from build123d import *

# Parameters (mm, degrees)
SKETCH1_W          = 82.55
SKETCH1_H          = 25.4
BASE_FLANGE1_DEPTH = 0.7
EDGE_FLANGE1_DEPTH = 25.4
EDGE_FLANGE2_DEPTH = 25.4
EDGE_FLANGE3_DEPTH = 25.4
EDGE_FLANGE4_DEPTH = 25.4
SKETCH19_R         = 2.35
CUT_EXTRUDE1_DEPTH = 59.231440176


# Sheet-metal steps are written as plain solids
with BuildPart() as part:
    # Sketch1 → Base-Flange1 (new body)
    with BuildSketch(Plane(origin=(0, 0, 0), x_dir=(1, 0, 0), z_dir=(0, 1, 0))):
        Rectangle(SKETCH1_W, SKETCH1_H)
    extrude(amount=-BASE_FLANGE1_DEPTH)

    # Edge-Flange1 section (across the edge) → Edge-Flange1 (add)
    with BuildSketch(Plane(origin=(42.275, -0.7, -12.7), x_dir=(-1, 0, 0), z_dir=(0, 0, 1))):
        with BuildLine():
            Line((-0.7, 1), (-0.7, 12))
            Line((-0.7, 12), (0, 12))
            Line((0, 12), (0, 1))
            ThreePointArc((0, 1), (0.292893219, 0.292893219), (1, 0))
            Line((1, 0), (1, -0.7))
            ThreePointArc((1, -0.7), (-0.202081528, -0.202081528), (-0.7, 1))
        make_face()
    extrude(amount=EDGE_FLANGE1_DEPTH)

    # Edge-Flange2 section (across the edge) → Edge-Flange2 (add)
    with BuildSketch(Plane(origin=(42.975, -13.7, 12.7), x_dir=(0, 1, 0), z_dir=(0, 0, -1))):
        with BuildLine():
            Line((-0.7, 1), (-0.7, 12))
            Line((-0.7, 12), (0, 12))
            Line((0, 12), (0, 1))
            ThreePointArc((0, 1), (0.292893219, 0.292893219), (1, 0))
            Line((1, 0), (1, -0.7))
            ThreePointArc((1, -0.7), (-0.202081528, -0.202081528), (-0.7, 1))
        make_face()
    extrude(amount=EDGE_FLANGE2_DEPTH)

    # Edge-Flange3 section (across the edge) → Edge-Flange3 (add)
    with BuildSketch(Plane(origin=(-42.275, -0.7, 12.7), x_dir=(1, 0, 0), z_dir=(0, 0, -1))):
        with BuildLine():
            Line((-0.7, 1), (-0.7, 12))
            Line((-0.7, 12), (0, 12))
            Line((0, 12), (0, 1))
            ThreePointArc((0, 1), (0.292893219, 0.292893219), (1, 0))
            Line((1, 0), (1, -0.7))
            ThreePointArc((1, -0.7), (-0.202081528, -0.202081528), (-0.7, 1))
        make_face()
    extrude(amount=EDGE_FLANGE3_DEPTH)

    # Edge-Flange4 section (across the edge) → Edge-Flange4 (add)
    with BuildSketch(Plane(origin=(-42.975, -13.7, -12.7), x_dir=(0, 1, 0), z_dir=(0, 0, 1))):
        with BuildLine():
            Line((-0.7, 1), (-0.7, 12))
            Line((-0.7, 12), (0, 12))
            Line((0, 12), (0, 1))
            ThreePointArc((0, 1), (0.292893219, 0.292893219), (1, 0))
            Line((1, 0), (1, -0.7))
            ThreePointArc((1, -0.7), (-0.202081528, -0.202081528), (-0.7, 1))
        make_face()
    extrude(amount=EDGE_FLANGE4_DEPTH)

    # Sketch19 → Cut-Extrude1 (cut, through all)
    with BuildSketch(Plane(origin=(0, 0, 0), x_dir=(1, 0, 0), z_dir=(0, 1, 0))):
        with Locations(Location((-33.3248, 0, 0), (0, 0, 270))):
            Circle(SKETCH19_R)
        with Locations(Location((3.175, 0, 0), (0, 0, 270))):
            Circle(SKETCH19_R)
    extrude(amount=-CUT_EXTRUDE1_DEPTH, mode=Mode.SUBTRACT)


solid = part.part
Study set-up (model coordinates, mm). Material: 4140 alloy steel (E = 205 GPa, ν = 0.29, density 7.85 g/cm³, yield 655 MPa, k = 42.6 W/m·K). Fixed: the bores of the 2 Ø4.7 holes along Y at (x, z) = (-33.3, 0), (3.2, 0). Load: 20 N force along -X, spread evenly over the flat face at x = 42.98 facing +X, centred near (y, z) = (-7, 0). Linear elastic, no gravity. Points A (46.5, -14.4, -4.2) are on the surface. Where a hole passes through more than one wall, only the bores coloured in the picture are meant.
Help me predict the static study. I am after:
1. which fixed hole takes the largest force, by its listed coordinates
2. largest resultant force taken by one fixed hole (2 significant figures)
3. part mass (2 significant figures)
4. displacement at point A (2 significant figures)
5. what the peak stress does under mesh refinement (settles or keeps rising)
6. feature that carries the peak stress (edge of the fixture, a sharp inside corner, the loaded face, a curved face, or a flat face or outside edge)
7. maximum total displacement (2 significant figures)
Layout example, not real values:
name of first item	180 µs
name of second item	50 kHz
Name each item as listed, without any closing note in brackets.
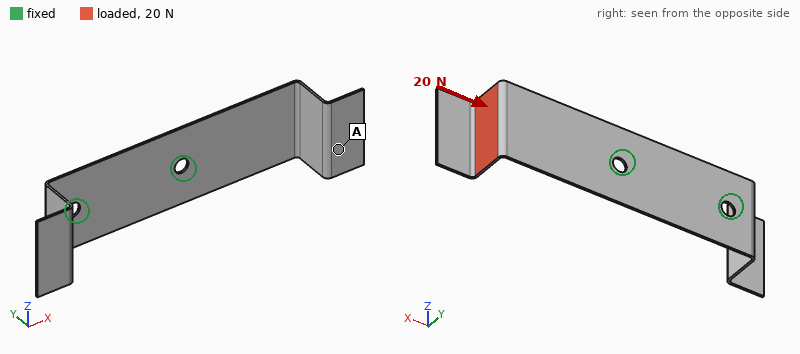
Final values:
which fixed hole takes the largest force, by its listed coordinates	(3.2, 0)
largest resultant force taken by one fixed hole	17 N
part mass	19 g
displacement at point A	0.96 mm
what the peak stress does under mesh refinement	keeps rising
feature that carries the peak stress	edge of the fixture
maximum total displacement	1.2 mm
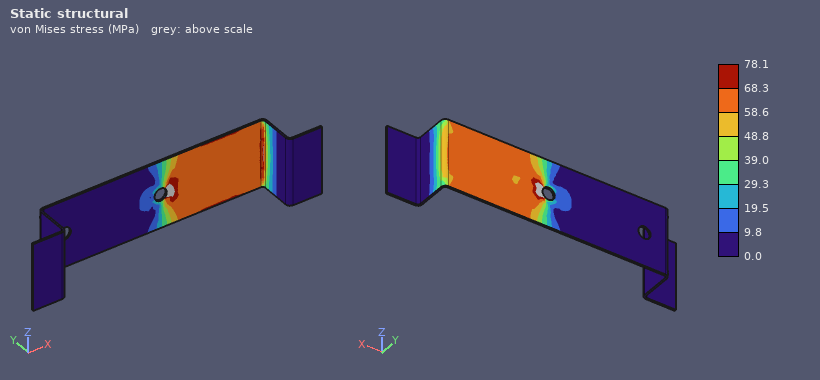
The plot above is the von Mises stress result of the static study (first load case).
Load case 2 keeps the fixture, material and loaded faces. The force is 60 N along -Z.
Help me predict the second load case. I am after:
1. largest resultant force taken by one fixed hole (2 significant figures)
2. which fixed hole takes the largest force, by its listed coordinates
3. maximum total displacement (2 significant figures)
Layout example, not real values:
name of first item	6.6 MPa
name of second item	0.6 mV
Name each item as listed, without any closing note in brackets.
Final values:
largest resultant force taken by one fixed hole	110 N
which fixed hole takes the largest force, by its listed coordinates	(3.2, 0)
maximum total displacement	1.2 mm
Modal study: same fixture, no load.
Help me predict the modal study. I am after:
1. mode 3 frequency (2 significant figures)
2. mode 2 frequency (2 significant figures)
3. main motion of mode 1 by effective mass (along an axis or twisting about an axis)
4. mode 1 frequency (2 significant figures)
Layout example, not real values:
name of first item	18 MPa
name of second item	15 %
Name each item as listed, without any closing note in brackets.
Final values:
mode 3 frequency	690 Hz
mode 2 frequency	490 Hz
main motion of mode 1 by effective mass	along Y
mode 1 frequency	180 Hz
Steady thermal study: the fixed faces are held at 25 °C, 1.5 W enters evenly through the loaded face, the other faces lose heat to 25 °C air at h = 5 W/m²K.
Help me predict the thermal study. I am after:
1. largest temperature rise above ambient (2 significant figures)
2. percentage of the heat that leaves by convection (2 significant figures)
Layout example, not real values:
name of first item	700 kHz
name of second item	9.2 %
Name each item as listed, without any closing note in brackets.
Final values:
largest temperature rise above ambient	63 K
percentage of the heat that leaves by convection	41 %
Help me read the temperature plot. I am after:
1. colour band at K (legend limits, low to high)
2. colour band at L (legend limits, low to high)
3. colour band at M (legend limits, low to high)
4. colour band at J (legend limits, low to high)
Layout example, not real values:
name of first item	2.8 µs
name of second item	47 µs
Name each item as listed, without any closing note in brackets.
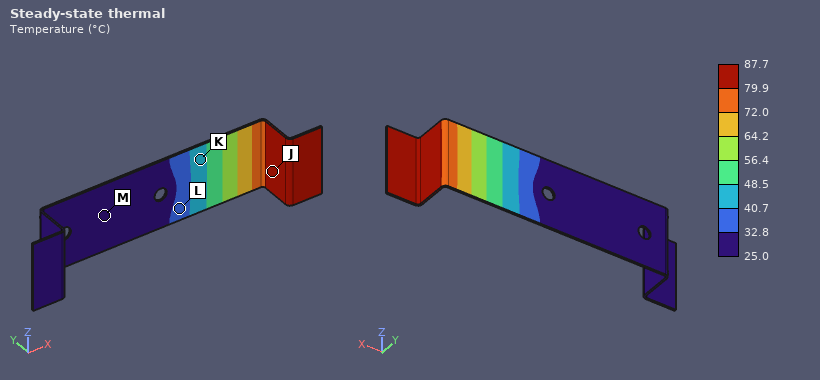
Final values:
colour band at K	40.7 to 48.5 °C
colour band at L	32.8 to 40.7 °C
colour band at M	25.0 to 32.8 °C
colour band at J	79.9 to 87.7 °C
